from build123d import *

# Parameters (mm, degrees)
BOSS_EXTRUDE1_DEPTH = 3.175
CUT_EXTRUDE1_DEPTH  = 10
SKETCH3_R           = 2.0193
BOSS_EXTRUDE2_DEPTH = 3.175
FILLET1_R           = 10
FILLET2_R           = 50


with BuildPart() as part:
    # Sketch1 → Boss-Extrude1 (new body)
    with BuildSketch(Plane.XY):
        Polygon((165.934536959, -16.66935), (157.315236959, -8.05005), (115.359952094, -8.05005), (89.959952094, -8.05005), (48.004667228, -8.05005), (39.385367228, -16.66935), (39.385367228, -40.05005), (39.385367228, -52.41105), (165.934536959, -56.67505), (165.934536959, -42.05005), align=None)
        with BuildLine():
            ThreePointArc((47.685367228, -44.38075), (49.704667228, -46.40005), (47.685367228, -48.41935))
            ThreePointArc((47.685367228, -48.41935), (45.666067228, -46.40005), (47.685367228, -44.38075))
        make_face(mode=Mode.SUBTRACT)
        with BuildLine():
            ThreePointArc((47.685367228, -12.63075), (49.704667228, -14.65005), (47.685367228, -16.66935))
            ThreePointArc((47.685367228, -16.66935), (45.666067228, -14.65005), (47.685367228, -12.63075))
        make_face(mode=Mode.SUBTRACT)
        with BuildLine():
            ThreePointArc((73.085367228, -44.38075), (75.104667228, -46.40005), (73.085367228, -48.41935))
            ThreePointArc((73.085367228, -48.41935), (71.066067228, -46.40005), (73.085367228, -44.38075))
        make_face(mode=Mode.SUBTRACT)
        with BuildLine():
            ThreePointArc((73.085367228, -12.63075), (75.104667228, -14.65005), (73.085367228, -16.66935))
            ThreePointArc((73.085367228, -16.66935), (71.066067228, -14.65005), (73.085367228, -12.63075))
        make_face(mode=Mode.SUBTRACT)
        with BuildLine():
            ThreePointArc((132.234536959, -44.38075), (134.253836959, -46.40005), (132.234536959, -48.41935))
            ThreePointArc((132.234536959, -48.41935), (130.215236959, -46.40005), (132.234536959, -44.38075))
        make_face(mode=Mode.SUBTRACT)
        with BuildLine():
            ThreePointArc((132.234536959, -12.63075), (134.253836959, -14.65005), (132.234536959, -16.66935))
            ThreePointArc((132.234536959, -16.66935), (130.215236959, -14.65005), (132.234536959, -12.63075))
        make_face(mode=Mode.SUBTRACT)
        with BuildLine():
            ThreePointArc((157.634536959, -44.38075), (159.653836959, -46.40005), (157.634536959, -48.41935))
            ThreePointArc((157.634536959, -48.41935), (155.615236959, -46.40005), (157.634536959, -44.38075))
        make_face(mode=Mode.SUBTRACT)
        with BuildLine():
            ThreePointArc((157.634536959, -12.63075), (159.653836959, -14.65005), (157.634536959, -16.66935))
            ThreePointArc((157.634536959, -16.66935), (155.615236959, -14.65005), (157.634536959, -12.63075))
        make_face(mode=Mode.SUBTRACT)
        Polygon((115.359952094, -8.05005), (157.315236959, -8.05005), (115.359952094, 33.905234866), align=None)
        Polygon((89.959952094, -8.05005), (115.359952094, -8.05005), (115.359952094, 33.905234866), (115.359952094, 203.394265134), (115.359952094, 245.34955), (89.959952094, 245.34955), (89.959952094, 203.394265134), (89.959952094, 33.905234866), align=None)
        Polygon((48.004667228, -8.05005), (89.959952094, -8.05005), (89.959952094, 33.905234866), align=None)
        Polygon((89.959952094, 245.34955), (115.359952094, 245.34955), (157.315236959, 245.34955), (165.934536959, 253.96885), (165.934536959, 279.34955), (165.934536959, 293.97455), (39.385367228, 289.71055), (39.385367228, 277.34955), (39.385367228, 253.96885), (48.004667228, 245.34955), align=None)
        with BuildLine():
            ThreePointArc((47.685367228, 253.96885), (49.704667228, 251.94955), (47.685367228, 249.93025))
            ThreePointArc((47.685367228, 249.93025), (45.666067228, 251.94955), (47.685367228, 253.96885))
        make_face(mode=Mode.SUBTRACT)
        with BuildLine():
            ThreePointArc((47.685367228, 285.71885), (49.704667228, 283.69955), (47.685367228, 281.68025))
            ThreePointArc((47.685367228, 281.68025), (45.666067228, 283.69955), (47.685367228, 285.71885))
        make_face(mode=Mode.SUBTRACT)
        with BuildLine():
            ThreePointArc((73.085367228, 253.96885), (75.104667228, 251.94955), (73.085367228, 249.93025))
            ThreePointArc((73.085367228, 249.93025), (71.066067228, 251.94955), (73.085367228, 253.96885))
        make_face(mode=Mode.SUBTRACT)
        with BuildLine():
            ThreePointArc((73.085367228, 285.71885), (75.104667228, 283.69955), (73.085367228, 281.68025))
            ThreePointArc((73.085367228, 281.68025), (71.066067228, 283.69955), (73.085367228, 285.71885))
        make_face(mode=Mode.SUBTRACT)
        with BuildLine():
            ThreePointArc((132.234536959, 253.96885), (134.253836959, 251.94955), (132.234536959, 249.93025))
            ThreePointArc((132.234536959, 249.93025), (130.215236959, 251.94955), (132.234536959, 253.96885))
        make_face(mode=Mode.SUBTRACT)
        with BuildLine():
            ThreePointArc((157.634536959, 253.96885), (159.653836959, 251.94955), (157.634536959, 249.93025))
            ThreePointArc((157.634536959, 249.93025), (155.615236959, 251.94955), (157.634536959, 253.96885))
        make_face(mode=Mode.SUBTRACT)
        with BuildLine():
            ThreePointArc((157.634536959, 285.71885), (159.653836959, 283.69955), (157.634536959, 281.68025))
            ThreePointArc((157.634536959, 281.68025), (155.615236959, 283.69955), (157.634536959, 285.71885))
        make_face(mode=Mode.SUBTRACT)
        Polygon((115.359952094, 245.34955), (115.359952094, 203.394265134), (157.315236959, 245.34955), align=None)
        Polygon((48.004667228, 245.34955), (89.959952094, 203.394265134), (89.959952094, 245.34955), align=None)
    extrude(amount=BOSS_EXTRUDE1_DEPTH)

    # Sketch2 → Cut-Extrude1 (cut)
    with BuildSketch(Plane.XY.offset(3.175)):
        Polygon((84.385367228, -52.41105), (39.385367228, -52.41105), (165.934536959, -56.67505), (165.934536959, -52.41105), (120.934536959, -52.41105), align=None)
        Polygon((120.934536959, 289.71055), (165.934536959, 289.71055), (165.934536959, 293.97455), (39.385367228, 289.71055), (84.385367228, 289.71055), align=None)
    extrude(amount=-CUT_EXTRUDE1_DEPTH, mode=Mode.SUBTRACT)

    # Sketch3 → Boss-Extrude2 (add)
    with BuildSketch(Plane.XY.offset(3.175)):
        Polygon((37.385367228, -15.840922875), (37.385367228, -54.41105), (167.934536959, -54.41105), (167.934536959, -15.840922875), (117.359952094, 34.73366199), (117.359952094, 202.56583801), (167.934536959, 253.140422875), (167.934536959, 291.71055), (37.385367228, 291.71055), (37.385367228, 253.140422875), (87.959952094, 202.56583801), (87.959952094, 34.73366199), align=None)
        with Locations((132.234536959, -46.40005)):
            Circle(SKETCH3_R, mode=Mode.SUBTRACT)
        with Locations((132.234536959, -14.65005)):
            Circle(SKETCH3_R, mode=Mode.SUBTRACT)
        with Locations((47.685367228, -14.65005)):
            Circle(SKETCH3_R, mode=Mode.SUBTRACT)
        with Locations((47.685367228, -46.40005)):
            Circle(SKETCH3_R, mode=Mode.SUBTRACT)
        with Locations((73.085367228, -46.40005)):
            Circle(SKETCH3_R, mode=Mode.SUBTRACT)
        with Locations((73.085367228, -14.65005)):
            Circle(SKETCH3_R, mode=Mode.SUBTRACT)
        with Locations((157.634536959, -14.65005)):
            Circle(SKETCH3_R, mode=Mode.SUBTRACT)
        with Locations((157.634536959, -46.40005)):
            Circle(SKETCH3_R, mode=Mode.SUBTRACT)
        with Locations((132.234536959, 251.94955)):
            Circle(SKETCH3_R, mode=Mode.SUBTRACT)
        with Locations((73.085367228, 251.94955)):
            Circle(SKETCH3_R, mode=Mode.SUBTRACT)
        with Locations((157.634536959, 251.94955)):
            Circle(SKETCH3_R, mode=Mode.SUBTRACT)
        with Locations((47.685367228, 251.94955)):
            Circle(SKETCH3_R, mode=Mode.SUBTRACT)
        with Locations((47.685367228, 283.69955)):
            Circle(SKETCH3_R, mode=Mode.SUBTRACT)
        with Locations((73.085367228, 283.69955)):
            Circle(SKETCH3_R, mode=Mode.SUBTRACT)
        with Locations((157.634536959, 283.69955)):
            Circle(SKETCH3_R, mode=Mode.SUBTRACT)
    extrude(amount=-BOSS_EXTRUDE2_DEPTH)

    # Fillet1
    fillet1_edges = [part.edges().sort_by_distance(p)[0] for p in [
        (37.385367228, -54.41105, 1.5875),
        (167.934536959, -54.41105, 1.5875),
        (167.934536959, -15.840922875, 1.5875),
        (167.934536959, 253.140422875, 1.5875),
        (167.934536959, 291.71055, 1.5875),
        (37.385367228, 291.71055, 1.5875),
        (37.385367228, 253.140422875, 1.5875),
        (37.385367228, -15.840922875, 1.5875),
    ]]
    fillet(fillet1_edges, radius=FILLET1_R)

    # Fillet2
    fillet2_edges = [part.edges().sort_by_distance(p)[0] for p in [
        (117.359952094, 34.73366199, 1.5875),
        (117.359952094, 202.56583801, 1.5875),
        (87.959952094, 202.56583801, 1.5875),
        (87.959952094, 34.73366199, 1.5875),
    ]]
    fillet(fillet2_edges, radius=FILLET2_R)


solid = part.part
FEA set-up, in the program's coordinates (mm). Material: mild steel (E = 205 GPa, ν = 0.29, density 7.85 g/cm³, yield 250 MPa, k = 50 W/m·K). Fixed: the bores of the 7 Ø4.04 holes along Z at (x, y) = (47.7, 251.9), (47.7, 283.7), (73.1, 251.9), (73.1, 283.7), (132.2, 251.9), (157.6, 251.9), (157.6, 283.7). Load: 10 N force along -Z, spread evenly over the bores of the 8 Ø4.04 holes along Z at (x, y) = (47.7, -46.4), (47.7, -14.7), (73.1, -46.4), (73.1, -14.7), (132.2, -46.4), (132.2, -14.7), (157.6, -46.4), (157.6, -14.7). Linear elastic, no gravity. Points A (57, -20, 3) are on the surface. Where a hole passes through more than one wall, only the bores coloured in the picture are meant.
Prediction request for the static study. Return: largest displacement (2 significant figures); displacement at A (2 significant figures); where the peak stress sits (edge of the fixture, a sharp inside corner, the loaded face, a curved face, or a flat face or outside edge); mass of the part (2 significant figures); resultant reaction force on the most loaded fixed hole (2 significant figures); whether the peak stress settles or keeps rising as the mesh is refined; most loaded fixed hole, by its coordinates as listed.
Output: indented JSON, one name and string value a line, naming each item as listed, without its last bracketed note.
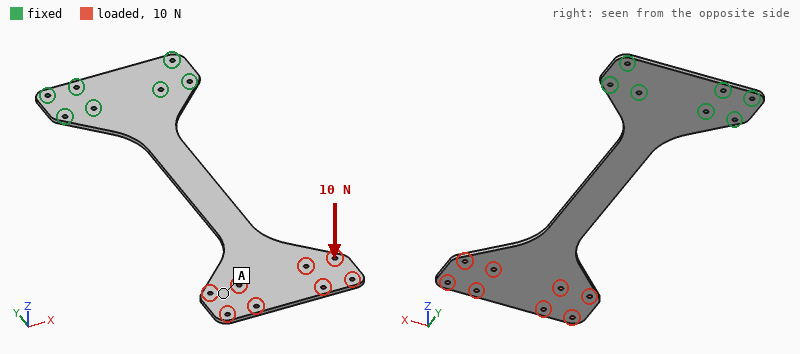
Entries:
{
  "largest displacement": "4.0 mm",
  "displacement at A": "3.3 mm",
  "where the peak stress sits": "edge of the fixture",
  "mass of the part": "570 g",
  "resultant reaction force on the most loaded fixed hole": "31 N",
  "whether the peak stress settles or keeps rising as the mesh is refined": "keeps rising",
  "most loaded fixed hole, by its coordinates as listed": "(73.1, 251.9)"
}
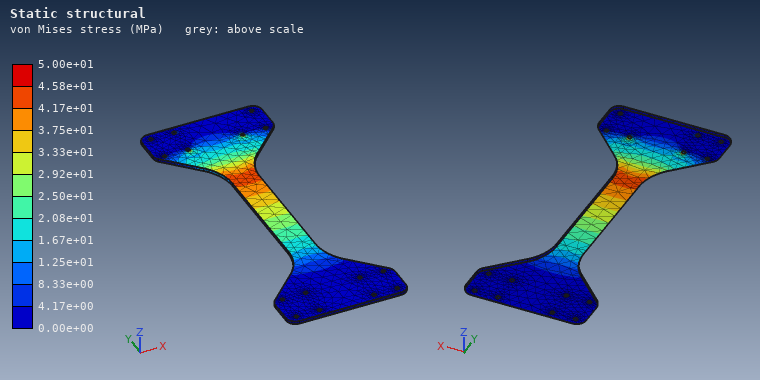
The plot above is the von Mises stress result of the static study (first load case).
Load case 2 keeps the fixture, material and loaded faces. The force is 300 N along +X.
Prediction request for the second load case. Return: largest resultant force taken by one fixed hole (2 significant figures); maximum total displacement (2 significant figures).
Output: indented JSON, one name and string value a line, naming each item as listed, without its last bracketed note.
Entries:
{
  "largest resultant force taken by one fixed hole": "760 N",
  "maximum total displacement": "1.2 mm"
}
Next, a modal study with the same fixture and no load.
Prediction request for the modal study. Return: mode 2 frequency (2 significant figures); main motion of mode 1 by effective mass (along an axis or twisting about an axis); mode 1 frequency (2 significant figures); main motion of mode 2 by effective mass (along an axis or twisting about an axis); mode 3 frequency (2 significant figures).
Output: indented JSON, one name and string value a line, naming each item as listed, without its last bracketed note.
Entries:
{
  "mode 2 frequency": "110 Hz",
  "main motion of mode 1 by effective mass": "along Z",
  "mode 1 frequency": "19 Hz",
  "main motion of mode 2 by effective mass": "twisting about Y",
  "mode 3 frequency": "170 Hz"
}
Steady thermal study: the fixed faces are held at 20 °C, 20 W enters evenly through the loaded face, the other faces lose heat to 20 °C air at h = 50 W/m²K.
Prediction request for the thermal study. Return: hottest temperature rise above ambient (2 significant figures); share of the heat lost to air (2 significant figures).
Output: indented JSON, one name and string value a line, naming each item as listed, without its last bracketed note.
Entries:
{
  "hottest temperature rise above ambient": "33 K",
  "share of the heat lost to air": "100 %"
}
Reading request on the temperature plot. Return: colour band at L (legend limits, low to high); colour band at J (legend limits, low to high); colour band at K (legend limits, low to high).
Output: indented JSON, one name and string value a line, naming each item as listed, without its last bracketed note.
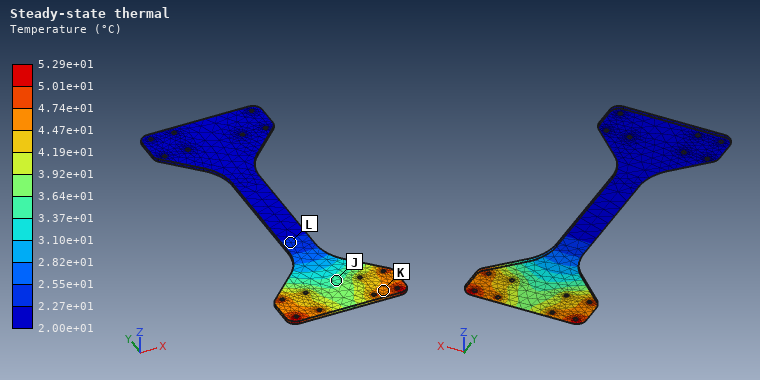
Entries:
{
  "colour band at L": "2.27e+01 to 2.55e+01 °C",
  "colour band at J": "3.37e+01 to 3.64e+01 °C",
  "colour band at K": "4.47e+01 to 4.74e+01 °C"
}
